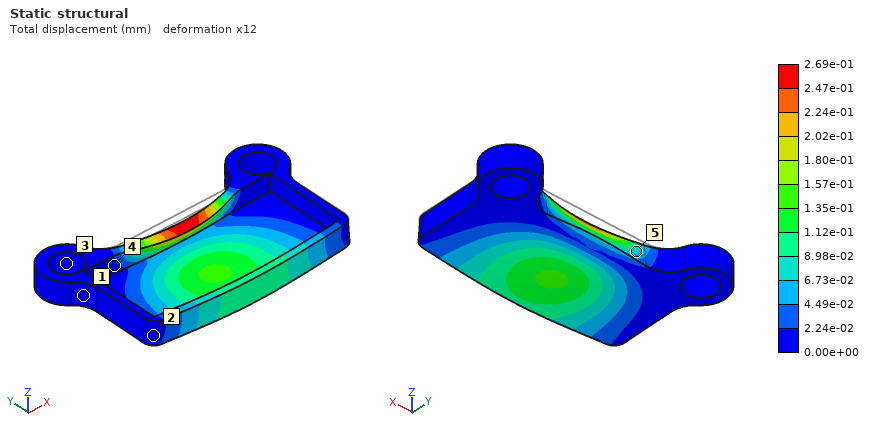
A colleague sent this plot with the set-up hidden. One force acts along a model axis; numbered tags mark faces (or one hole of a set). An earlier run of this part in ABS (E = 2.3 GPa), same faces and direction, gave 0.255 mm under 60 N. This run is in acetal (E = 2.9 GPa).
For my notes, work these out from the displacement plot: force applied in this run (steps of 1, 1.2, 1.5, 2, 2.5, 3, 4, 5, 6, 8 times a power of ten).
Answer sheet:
80 N
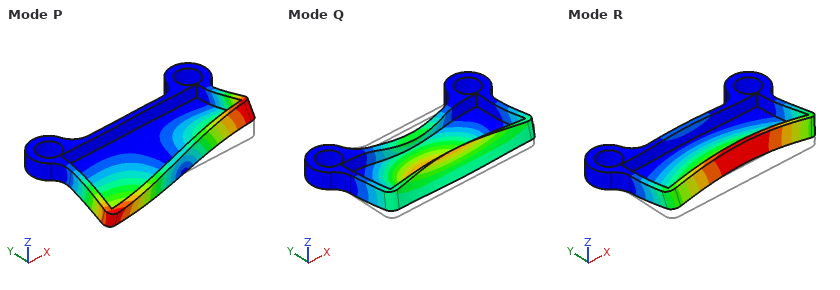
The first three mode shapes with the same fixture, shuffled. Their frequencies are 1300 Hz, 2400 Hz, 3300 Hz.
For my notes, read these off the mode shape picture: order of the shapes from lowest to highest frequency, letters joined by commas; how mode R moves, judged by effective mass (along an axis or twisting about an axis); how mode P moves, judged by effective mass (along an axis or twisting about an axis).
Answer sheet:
R, P, Q
along Z
twisting about Y
